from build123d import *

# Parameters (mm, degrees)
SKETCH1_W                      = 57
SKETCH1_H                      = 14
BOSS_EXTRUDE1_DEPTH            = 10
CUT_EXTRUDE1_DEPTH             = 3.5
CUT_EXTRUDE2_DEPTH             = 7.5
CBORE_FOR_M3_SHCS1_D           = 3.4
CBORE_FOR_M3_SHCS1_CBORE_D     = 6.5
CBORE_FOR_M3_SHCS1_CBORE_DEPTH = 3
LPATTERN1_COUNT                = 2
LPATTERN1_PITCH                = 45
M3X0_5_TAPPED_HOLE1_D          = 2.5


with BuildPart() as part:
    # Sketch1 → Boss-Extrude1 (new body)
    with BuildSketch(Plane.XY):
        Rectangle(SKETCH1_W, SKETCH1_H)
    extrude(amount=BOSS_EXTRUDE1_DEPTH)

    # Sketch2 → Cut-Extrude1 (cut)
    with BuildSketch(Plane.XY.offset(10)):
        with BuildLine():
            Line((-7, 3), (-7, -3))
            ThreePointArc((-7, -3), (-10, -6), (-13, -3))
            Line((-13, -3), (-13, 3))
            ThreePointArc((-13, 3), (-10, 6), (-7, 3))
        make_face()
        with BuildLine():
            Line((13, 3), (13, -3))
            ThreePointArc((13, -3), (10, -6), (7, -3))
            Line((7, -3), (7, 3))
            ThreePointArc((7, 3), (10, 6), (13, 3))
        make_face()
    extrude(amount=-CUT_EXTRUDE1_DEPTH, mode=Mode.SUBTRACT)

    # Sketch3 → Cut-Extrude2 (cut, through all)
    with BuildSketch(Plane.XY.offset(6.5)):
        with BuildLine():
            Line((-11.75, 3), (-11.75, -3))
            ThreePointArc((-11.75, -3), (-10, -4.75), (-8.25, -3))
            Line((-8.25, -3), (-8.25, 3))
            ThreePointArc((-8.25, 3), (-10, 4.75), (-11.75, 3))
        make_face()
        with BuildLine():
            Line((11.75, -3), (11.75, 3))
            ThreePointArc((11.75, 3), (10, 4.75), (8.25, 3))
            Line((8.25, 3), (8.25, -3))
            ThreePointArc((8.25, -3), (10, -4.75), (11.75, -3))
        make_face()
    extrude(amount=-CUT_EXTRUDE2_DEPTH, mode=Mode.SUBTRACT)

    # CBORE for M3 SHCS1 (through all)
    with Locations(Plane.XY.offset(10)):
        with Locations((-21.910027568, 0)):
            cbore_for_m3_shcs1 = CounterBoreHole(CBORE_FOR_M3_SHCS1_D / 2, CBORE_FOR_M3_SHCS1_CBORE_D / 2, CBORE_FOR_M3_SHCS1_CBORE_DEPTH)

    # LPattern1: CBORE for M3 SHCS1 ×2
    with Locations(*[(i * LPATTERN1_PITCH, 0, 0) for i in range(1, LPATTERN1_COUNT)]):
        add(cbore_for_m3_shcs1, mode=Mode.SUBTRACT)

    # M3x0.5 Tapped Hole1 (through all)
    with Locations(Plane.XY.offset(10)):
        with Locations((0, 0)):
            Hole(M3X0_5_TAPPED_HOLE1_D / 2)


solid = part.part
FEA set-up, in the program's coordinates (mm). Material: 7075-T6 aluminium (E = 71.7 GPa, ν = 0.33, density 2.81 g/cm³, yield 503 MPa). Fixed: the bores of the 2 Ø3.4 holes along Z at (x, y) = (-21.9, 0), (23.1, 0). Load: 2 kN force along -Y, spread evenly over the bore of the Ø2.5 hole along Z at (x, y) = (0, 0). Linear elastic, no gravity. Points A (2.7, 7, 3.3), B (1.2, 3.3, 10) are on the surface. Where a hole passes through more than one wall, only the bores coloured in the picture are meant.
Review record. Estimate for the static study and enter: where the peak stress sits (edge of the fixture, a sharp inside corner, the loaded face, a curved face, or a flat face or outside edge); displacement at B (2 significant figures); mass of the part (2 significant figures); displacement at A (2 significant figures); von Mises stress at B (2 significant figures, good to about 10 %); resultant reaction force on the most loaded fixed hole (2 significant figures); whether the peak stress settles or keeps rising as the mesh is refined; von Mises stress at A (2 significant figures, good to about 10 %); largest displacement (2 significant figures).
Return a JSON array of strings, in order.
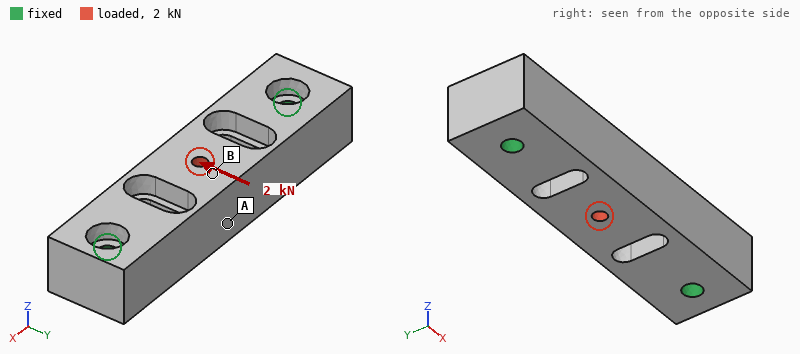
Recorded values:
["edge of the fixture", "41 µm", "19 g", "35 µm", "16 MPa", "1.0 kN", "keeps rising", "59 MPa", "41 µm"]
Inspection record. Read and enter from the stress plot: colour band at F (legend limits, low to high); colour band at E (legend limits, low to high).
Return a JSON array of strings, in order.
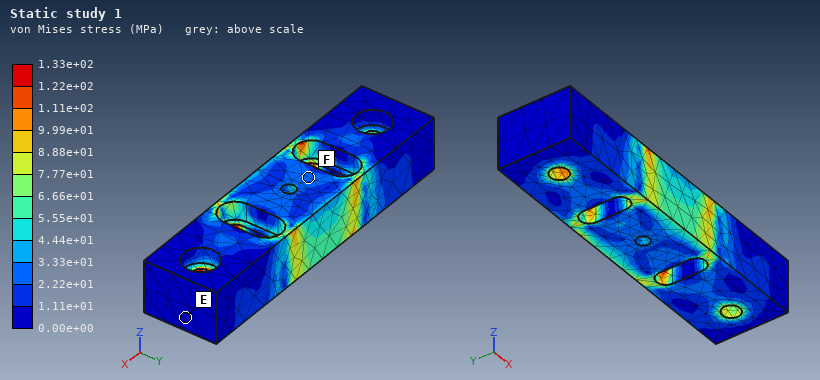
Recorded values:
["2.22e+01 to 3.33e+01 MPa", "0.00e+00 to 1.11e+01 MPa"]
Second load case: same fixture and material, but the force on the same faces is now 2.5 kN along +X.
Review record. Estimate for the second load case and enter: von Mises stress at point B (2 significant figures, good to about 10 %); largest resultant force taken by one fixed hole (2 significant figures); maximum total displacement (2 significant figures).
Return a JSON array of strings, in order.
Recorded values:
["17 MPa", "1.3 kN", "9.2 µm"]
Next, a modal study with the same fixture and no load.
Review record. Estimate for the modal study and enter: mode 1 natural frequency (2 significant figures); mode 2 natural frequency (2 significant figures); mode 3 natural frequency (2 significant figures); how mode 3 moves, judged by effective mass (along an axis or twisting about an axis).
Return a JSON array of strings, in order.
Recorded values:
["15 kHz", "15 kHz", "23 kHz", "twisting about X"]
